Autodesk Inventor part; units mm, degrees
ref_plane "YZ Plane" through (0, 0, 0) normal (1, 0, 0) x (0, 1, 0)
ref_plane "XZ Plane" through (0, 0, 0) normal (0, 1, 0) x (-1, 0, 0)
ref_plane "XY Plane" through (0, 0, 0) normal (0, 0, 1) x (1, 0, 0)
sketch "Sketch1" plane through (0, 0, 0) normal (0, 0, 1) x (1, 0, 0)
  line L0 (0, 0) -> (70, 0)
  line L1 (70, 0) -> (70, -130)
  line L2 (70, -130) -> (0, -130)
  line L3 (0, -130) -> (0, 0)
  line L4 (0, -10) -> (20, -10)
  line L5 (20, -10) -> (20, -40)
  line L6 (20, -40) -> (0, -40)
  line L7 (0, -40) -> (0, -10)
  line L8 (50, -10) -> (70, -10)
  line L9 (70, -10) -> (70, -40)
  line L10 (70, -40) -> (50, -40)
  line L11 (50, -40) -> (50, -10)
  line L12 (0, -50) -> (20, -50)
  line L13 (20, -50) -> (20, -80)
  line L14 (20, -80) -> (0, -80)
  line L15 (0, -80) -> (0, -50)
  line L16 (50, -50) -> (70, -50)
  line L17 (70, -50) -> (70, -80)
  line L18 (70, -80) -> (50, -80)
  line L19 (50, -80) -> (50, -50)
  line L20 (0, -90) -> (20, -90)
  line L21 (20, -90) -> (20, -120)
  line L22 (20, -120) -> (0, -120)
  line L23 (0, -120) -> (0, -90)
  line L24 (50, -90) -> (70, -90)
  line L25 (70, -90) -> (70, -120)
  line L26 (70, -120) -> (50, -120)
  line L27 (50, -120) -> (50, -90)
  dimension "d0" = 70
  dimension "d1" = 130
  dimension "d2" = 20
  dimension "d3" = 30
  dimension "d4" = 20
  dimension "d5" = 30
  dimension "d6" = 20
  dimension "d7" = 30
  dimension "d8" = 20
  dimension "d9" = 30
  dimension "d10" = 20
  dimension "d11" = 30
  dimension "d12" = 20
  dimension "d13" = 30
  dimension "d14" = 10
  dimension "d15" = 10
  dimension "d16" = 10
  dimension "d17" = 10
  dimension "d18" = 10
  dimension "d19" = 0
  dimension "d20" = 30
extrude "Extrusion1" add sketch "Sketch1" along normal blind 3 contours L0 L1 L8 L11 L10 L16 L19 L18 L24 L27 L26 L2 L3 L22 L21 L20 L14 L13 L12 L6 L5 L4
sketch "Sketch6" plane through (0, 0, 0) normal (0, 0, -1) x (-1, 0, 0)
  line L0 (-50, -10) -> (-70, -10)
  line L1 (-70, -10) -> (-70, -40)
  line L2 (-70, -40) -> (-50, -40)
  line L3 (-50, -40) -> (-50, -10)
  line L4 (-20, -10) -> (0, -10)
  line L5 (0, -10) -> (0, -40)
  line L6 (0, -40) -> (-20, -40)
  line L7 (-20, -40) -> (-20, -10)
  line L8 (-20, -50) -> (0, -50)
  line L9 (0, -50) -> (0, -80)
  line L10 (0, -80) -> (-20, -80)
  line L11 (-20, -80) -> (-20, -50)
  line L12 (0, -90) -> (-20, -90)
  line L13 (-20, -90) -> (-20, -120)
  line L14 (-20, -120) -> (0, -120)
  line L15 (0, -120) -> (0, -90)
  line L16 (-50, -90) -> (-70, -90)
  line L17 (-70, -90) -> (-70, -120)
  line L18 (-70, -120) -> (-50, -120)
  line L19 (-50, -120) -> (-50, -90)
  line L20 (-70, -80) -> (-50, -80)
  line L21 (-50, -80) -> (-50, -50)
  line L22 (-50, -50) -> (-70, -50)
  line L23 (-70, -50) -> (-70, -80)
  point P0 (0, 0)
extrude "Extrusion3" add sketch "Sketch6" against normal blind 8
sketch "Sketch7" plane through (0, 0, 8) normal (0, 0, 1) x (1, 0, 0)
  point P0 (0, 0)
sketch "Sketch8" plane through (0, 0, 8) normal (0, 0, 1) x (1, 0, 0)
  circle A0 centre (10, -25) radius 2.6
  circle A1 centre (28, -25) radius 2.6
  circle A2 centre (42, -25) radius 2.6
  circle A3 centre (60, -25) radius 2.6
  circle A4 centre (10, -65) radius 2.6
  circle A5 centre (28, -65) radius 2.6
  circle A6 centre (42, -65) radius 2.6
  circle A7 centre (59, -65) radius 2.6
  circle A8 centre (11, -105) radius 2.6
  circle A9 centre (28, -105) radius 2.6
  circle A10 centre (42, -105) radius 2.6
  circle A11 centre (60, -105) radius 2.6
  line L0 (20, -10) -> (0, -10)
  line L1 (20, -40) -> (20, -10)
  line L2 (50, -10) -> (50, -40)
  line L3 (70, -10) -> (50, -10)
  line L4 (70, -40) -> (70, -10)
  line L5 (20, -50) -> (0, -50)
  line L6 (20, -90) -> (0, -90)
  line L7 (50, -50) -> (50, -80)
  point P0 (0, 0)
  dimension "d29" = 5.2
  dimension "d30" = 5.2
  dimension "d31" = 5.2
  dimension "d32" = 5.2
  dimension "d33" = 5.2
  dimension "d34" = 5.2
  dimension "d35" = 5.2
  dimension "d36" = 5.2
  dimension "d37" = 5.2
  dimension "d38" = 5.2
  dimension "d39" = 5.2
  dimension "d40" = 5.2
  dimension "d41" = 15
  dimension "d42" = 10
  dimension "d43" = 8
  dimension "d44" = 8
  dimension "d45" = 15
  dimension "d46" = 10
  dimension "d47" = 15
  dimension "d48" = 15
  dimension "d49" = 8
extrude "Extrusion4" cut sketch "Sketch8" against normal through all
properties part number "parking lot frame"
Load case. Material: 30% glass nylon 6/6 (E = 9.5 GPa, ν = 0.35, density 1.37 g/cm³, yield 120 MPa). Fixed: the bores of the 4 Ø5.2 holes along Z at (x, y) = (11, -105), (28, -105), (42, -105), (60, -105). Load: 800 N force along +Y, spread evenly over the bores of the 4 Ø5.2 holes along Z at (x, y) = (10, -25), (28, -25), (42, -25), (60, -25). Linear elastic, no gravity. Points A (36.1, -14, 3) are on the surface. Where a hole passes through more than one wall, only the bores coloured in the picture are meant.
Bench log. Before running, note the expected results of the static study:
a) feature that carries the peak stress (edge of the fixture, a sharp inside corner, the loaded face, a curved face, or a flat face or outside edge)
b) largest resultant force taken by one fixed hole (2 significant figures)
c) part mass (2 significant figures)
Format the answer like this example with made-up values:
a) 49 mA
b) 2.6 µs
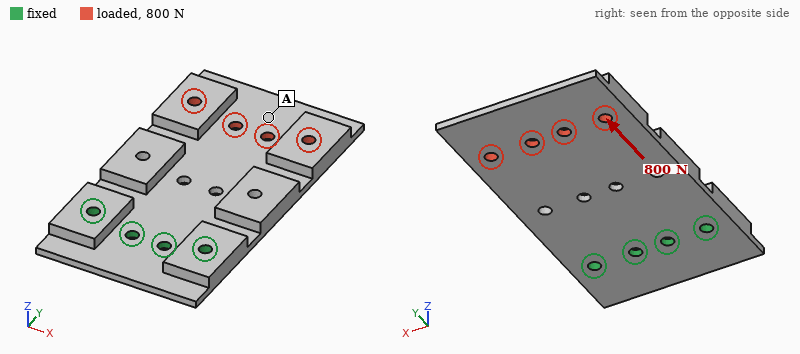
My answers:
a) a flat face or outside edge
b) 310 N
c) 60 g
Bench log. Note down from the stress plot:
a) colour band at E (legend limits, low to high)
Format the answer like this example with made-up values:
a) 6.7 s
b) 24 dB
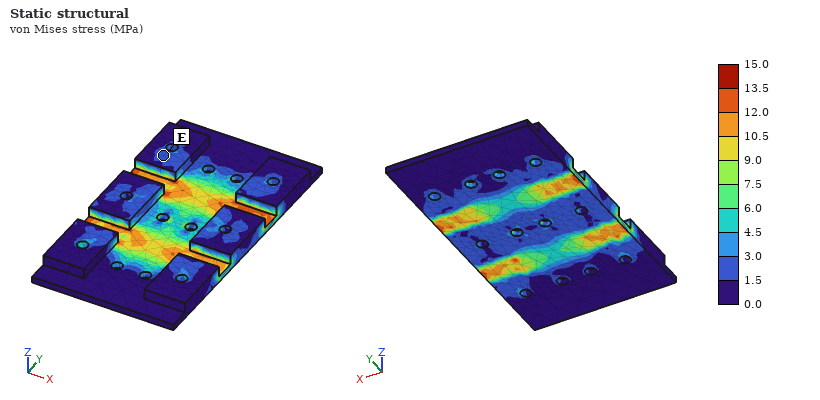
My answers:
a) 1.5 to 3.0 MPa
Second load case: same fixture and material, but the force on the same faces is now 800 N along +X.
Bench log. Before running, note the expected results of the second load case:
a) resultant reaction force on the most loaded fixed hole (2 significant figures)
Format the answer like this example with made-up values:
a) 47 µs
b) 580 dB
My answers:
a) 1.2 kN
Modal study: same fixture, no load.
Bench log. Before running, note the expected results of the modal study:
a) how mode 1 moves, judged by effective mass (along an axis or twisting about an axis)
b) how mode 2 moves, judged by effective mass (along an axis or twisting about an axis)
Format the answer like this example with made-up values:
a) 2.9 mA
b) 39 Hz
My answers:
a) along Z
b) twisting about Y
